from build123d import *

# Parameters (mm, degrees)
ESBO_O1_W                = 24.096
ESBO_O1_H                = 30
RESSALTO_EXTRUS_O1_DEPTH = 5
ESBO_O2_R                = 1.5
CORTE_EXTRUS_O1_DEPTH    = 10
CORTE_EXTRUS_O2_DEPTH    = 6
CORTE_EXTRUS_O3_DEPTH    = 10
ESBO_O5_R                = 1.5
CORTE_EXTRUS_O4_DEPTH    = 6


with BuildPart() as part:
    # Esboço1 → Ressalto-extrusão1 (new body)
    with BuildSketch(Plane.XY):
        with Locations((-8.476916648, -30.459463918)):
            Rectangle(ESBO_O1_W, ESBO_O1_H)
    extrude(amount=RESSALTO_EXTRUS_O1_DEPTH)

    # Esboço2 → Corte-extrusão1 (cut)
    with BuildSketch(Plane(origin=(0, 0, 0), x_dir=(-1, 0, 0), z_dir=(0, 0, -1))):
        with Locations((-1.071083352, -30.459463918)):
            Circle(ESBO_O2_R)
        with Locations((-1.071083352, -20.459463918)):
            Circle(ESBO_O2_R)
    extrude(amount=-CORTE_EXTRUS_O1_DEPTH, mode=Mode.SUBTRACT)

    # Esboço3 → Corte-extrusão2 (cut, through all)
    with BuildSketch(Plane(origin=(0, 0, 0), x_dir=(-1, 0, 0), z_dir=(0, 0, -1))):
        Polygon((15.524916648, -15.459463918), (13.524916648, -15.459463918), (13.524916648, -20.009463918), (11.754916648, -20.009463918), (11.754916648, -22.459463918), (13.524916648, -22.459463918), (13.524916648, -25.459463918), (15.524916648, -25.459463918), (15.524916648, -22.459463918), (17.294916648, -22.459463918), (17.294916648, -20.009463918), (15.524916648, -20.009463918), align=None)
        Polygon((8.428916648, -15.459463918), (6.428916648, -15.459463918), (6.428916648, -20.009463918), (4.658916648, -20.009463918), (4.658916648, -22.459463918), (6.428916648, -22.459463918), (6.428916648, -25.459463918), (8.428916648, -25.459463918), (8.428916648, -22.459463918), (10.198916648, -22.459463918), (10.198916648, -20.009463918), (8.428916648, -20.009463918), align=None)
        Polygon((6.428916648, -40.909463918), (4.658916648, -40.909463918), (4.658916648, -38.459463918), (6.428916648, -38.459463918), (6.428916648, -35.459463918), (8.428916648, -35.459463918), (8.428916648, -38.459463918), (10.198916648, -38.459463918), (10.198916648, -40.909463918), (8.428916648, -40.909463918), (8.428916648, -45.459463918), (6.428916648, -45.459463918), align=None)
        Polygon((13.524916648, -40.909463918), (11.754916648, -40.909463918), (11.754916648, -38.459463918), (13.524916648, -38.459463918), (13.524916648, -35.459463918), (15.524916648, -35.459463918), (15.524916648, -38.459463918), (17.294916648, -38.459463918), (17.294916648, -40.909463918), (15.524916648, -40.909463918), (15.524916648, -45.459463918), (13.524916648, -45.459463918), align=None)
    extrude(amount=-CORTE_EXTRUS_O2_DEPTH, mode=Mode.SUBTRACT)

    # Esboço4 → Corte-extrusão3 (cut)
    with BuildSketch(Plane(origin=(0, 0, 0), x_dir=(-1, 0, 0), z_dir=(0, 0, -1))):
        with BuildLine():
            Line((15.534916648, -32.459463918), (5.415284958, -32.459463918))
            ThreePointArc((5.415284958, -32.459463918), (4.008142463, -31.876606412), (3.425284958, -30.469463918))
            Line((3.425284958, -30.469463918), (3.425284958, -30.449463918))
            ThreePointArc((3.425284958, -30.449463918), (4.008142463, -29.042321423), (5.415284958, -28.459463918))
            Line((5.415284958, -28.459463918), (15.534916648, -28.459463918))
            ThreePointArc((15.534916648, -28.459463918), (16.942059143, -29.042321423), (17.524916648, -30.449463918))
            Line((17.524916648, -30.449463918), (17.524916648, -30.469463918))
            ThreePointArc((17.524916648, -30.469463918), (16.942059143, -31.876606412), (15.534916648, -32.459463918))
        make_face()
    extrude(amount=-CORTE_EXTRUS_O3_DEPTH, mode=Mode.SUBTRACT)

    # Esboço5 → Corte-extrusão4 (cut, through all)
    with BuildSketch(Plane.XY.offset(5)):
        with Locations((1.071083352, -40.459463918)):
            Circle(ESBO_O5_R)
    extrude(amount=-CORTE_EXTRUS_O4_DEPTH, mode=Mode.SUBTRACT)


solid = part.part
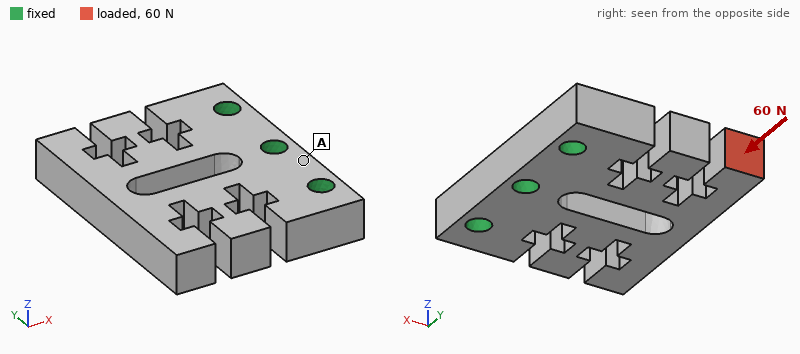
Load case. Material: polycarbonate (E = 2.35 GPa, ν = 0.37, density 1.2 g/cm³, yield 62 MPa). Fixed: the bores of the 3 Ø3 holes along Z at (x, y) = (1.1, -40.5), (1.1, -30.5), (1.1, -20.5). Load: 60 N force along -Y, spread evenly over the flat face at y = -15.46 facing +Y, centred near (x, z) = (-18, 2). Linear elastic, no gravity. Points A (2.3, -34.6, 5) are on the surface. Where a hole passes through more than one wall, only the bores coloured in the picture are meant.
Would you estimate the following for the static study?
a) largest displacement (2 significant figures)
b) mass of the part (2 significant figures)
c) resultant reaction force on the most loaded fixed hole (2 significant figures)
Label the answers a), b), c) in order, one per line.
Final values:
a) 0.34 mm
b) 3.2 g
c) 64 N
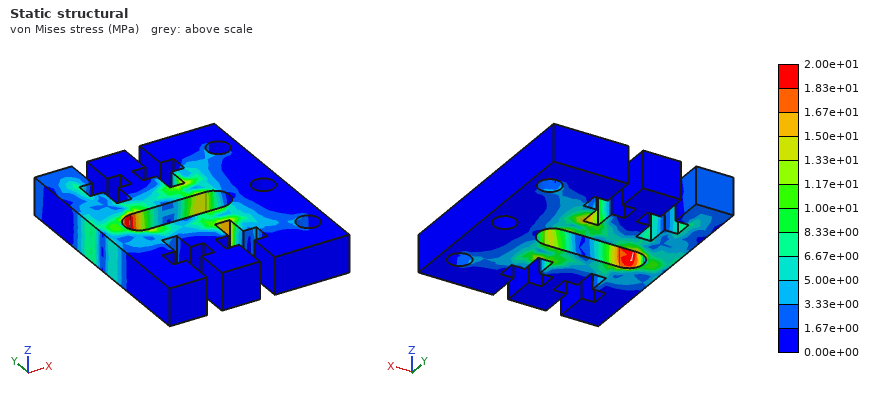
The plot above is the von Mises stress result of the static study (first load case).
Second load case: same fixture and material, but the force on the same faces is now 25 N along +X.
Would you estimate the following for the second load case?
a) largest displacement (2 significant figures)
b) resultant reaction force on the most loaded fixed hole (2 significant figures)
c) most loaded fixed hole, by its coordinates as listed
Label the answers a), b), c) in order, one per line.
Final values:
a) 0.39 mm
b) 35 N
c) (1.1, -30.5)
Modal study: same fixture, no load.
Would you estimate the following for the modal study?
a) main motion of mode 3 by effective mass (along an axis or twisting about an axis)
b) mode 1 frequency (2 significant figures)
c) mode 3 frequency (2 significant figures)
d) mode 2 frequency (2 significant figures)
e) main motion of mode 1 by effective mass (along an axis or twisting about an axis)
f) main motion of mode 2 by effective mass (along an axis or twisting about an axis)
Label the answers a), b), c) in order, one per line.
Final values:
a) along Y
b) 1600 Hz
c) 2000 Hz
d) 1700 Hz
e) along Z
f) twisting about X
